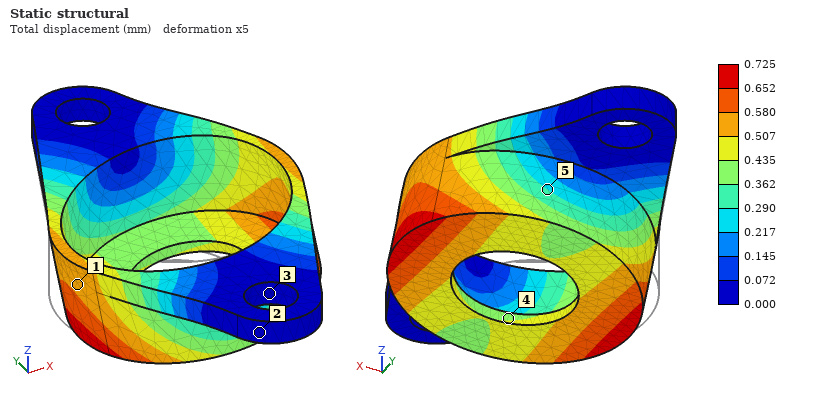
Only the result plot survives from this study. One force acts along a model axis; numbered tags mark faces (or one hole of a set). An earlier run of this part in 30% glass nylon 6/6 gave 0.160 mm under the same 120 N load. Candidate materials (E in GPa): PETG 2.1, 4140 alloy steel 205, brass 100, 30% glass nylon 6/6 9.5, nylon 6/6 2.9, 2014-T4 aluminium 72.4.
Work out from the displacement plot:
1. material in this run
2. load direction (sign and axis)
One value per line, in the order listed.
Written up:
PETG
+X
